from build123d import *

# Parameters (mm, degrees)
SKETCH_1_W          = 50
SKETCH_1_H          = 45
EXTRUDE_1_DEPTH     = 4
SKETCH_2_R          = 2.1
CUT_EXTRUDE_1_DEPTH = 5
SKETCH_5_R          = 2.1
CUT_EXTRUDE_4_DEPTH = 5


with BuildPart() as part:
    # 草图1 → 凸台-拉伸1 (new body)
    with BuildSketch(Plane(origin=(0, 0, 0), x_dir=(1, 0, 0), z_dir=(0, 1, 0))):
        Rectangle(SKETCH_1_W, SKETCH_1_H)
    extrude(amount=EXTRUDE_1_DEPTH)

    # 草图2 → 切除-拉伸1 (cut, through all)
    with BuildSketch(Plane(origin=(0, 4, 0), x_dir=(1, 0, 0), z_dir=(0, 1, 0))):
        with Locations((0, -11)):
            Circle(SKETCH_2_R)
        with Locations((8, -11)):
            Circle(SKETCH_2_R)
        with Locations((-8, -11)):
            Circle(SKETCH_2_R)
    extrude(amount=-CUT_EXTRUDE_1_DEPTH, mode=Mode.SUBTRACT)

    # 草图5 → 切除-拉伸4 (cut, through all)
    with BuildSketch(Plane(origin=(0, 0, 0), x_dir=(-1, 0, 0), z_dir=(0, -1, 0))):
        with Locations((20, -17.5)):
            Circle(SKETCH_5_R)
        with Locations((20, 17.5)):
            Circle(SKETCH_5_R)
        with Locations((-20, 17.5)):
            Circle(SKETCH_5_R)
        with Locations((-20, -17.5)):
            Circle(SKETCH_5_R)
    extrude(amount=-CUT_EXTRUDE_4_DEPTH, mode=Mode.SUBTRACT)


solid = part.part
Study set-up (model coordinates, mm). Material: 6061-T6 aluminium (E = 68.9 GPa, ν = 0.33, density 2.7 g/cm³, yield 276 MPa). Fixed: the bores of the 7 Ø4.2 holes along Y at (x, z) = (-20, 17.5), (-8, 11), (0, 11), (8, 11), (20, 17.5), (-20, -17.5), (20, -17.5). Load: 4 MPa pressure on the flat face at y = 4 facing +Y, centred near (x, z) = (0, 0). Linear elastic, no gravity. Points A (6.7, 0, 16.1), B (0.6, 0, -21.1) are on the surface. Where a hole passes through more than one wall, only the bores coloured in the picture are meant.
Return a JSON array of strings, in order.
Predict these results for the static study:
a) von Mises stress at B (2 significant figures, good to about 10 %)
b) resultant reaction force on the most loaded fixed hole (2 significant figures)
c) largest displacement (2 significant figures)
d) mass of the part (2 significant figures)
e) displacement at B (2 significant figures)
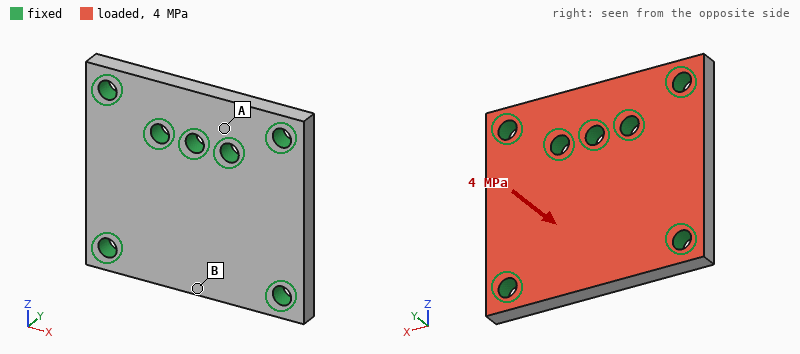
["91 MPa", "1.8 kN", "71 µm", "23 g", "68 µm"]
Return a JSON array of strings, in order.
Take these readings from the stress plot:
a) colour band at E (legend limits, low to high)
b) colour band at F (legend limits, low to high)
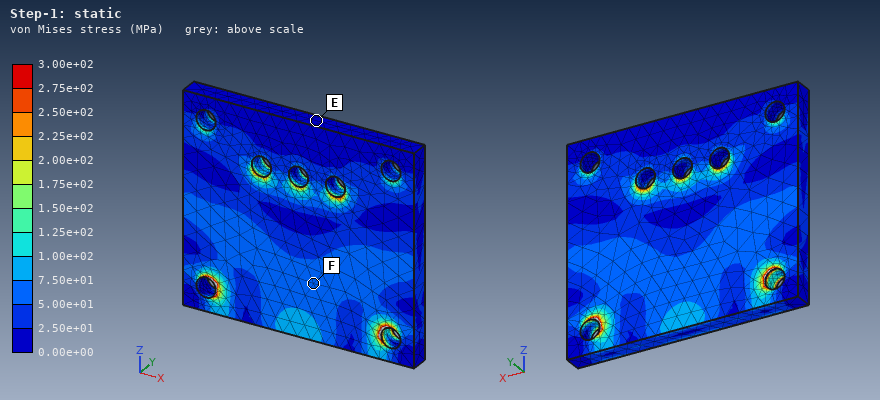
["0.00e+00 to 2.50e+01 MPa", "5.00e+01 to 7.50e+01 MPa"]
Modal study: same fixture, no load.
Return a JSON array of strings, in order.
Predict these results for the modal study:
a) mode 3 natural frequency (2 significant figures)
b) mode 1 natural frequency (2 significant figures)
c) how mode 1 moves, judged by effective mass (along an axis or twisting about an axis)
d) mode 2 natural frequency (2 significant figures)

["21 kHz", "14 kHz", "along Y", "20 kHz"]
